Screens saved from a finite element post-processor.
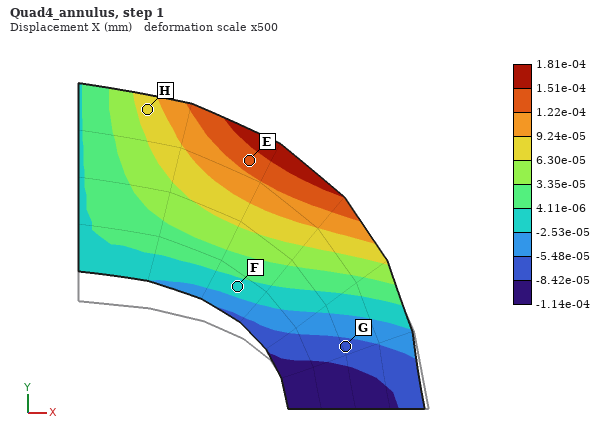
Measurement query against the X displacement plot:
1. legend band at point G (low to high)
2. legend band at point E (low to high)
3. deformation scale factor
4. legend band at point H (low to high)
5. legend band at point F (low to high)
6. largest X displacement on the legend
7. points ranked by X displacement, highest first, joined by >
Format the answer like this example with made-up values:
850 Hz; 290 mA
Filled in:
-8.42e-05 to -5.48e-05 mm; 1.22e-04 to 1.51e-04 mm; 500; 6.30e-05 to 9.24e-05 mm; -2.53e-05 to 4.11e-06 mm; 1.81e-04 mm; E > H > F > G
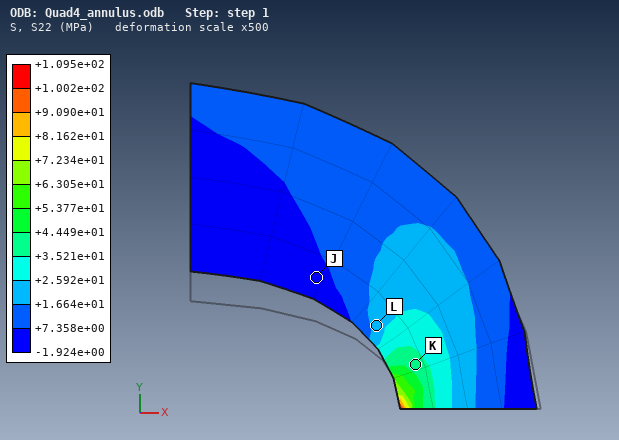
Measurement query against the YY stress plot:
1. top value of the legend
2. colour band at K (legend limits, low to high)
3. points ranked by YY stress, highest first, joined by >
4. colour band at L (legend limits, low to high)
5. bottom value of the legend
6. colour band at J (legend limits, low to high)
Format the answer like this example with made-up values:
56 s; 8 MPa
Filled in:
+1.095e+02 MPa; +3.521e+01 to +4.449e+01 MPa; K > L > J; +1.664e+01 to +2.592e+01 MPa; -1.924e+00 MPa; -1.924e+00 to +7.358e+00 MPa
